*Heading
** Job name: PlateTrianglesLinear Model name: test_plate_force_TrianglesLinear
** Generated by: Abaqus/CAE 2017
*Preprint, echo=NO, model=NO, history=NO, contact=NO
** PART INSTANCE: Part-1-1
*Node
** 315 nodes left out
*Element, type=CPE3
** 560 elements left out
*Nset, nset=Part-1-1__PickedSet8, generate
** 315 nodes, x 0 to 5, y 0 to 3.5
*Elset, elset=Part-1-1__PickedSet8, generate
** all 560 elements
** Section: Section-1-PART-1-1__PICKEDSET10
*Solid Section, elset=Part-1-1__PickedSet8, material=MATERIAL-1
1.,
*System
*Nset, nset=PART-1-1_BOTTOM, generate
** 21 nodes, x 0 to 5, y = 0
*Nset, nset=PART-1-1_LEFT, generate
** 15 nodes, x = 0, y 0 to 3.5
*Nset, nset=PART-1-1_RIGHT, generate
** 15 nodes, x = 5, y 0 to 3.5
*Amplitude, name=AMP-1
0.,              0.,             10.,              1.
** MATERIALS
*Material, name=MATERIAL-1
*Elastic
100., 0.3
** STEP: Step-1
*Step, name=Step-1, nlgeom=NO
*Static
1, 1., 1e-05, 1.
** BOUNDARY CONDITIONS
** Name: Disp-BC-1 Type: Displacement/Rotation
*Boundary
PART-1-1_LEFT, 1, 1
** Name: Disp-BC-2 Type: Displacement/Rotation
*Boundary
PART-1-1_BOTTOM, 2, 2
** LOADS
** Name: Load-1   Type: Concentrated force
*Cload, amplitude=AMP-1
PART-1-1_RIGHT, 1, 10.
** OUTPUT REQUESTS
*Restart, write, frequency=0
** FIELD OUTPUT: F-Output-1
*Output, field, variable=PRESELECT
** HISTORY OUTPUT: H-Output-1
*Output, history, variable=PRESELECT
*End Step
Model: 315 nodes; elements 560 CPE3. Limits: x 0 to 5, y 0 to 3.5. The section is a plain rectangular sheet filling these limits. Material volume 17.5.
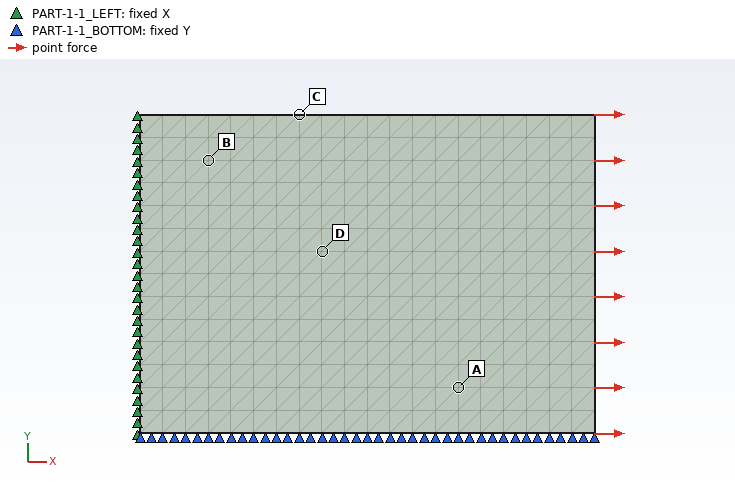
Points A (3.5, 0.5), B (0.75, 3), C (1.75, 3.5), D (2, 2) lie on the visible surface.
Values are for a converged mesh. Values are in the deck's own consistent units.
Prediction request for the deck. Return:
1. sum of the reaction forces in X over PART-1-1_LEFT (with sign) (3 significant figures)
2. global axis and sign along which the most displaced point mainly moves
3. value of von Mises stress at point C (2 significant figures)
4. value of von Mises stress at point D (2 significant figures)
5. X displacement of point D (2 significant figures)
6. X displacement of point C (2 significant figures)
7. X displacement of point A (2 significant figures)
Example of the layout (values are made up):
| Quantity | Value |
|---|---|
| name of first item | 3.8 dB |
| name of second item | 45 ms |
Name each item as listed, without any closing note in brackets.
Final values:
| Quantity | Value |
|---|---|
| sum of the reaction forces in X over PART-1-1_LEFT (with sign) | -15.0 |
| global axis and sign along which the most displaced point mainly moves | +X |
| value of von Mises stress at point C | 3.9 |
| value of von Mises stress at point D | 3.8 |
| X displacement of point D | 0.078 |
| X displacement of point C | 0.069 |
| X displacement of point A | 0.14 |
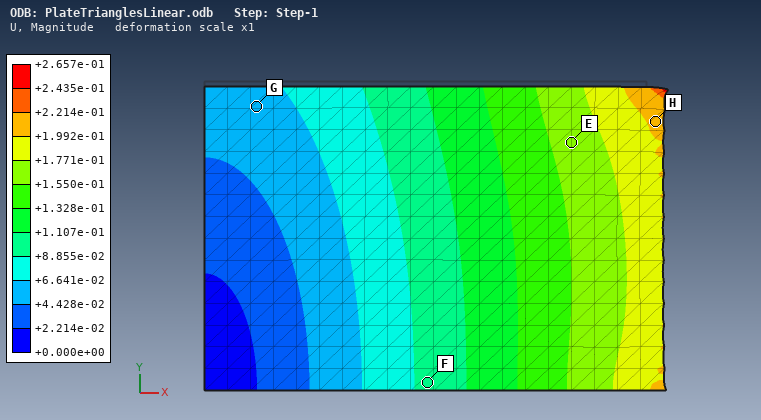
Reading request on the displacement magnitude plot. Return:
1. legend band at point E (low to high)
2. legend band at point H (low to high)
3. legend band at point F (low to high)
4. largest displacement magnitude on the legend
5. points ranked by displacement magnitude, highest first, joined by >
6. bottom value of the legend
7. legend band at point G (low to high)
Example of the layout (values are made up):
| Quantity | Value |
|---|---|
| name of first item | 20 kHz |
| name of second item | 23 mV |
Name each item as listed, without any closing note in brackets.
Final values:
| Quantity | Value |
|---|---|
| legend band at point E | +1.550e-01 to +1.771e-01 |
| legend band at point H | +1.992e-01 to +2.214e-01 |
| legend band at point F | +8.855e-02 to +1.107e-01 |
| largest displacement magnitude on the legend | +2.657e-01 |
| points ranked by displacement magnitude, highest first, joined by > | H > E > F > G |
| bottom value of the legend | +0.000e+00 |
| legend band at point G | +4.428e-02 to +6.641e-02 |
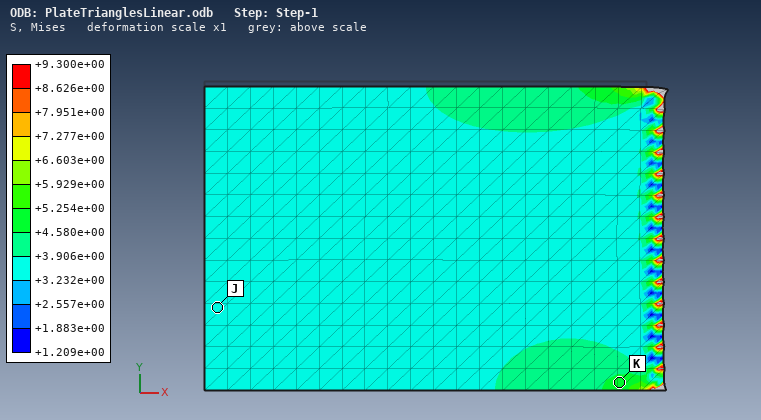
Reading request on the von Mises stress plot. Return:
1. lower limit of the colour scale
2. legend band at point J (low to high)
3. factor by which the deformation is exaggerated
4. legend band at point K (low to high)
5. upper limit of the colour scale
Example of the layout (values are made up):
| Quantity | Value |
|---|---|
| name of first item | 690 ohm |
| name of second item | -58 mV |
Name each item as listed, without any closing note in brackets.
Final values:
| Quantity | Value |
|---|---|
| lower limit of the colour scale | +1.209e+00 |
| legend band at point J | +3.232e+00 to +3.906e+00 |
| factor by which the deformation is exaggerated | 1 |
| legend band at point K | +4.580e+00 to +5.254e+00 |
| upper limit of the colour scale | +9.300e+00 |
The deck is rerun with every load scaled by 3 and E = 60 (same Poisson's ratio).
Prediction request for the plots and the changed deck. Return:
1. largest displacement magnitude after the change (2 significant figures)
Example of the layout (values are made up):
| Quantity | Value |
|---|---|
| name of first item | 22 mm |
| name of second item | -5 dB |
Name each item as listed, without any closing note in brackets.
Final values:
| Quantity | Value |
|---|---|
| largest displacement magnitude after the change | 1.3 |
